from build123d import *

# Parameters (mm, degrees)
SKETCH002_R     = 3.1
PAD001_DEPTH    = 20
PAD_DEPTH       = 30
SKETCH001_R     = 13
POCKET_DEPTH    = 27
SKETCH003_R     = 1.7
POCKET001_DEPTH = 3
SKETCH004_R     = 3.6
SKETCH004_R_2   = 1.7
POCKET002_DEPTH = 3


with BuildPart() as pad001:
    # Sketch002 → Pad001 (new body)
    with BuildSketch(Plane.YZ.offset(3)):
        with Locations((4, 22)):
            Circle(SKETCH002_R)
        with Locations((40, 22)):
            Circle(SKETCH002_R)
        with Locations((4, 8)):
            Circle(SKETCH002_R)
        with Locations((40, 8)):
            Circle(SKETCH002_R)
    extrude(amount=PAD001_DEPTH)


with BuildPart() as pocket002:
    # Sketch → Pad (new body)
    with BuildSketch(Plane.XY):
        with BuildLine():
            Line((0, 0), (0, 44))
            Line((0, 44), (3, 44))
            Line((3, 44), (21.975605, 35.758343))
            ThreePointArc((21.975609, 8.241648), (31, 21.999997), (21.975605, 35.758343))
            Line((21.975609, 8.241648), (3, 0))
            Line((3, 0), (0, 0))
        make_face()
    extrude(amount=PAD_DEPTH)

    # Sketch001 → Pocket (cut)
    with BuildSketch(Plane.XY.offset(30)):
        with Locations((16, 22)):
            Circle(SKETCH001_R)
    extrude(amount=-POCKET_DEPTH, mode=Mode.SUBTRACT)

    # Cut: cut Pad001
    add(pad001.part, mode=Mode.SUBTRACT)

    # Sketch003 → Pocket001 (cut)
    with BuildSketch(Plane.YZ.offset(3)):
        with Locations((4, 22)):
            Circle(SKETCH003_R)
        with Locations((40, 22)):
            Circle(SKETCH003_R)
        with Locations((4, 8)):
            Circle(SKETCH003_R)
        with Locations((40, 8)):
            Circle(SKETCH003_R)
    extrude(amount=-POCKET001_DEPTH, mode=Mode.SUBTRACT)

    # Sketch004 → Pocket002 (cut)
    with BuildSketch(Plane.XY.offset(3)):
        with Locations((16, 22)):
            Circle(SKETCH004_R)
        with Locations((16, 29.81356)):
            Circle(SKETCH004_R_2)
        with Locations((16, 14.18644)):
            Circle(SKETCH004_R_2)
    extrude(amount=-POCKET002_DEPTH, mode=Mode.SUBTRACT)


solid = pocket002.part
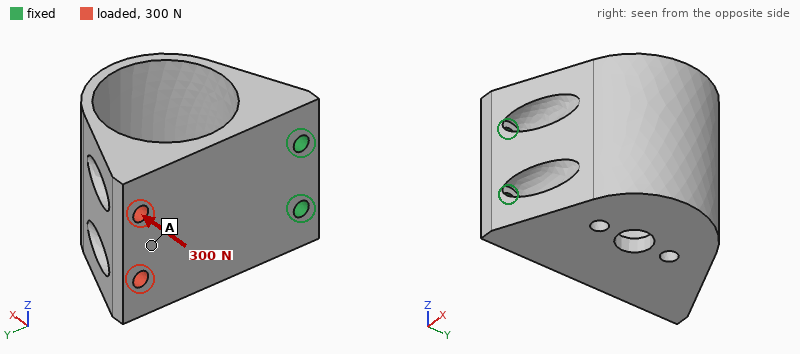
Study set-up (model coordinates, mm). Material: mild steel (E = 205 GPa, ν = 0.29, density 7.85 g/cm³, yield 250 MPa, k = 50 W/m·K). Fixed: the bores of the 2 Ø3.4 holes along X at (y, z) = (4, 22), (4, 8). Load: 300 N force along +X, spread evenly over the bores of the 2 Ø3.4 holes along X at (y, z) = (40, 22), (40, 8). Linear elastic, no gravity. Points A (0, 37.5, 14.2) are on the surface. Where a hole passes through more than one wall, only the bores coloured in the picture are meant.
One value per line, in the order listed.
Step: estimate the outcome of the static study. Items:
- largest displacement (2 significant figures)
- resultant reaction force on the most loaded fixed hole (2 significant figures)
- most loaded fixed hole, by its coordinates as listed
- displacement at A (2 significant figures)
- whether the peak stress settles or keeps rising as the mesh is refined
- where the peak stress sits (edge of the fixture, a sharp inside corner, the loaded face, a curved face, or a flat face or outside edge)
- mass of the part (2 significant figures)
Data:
57 µm
170 N
(4, 8)
46 µm
keeps rising
edge of the fixture
110 g
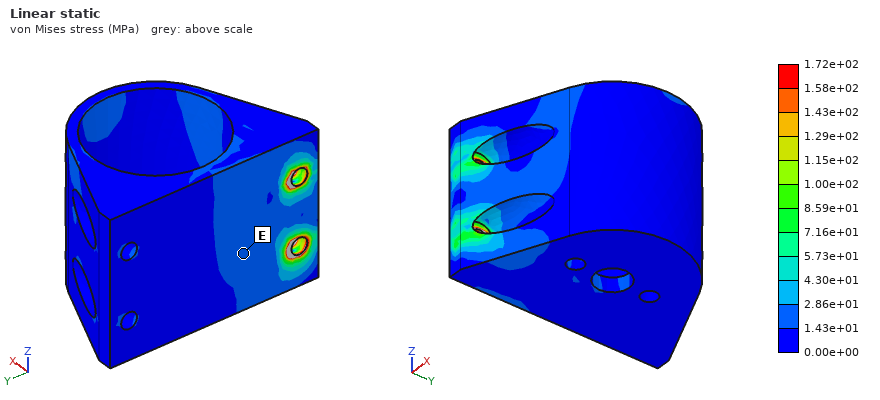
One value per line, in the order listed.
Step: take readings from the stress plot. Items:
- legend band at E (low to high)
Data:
1.43e+01 to 2.86e+01 MPa
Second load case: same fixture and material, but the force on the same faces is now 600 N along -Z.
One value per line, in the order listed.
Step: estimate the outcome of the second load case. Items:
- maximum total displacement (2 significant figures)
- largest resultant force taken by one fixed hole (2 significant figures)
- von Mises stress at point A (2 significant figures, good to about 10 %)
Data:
14 µm
1.3 kN
11 MPa
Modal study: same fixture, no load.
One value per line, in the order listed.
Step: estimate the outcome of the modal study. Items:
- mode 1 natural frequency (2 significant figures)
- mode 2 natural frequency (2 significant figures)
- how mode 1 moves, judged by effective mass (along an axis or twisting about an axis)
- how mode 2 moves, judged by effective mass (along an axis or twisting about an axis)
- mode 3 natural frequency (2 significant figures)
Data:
1700 Hz
5200 Hz
along X
along Z
7400 Hz
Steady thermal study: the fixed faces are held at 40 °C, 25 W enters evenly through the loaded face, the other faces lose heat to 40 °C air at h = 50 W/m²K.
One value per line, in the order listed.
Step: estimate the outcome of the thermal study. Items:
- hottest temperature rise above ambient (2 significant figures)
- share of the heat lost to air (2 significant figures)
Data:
82 K
50 %
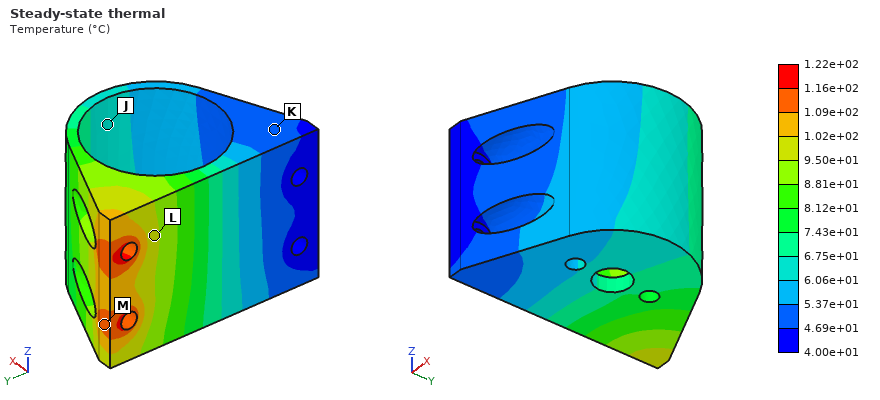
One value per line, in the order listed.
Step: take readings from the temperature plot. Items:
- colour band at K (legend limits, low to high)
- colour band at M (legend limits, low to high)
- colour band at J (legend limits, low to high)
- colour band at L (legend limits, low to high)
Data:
4.69e+01 to 5.37e+01 °C
1.09e+02 to 1.16e+02 °C
6.06e+01 to 6.75e+01 °C
9.50e+01 to 1.02e+02 °C
